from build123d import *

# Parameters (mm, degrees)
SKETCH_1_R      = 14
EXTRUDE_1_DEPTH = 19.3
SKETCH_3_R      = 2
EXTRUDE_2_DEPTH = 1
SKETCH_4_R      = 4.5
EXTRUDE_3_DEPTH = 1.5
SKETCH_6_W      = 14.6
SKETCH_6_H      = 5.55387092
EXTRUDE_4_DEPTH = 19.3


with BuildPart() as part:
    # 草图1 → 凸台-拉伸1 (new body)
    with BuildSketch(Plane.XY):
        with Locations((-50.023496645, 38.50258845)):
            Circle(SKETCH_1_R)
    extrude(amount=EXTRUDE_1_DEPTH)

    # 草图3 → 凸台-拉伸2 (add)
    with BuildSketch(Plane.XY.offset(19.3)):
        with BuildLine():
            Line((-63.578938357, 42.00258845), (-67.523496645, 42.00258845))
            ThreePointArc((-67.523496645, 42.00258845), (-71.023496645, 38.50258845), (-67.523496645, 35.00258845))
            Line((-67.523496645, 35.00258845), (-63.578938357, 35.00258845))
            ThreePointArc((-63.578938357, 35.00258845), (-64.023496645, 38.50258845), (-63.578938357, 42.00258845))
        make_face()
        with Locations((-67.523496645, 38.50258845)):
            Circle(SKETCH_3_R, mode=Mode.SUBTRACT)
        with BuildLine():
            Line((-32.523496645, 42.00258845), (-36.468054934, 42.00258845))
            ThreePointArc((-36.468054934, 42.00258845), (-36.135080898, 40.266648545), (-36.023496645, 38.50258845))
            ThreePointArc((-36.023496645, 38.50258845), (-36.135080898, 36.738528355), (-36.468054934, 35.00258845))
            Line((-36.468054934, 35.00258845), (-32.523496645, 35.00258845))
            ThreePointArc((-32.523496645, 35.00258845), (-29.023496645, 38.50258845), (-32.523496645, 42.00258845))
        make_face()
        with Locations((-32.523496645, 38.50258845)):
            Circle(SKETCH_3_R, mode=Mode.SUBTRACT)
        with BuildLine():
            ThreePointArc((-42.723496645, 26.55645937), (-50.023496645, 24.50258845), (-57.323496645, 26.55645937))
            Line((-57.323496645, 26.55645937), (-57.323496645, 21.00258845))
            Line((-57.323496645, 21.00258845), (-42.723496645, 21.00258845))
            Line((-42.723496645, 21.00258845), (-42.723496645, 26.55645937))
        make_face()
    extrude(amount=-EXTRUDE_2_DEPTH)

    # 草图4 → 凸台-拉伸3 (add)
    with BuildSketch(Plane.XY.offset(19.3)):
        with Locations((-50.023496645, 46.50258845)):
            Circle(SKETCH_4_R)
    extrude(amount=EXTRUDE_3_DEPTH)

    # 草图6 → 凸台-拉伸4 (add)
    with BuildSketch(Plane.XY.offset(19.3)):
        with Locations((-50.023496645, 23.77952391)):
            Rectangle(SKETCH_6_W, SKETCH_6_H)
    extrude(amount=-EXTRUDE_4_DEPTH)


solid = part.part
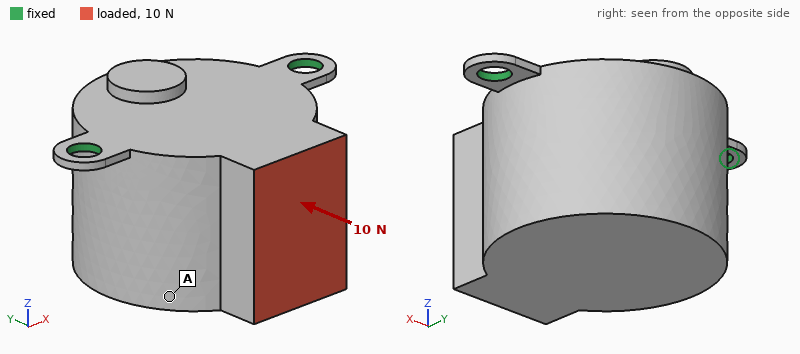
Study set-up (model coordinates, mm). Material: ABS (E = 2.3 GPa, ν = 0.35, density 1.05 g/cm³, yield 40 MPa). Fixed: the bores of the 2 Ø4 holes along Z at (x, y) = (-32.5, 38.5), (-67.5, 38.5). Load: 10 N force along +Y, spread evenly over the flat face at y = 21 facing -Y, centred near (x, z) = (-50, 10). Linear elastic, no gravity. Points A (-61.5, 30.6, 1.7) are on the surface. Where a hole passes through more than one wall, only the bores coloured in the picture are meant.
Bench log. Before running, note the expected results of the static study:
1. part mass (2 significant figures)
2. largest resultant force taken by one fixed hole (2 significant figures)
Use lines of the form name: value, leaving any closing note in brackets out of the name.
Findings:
part mass: 14 g
largest resultant force taken by one fixed hole: 5.0 N
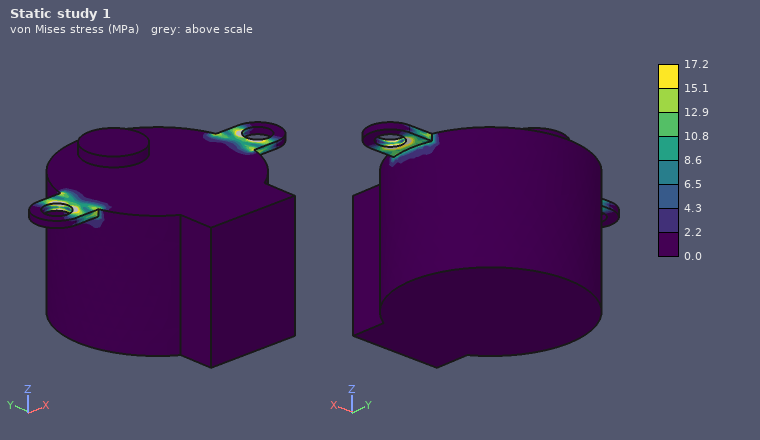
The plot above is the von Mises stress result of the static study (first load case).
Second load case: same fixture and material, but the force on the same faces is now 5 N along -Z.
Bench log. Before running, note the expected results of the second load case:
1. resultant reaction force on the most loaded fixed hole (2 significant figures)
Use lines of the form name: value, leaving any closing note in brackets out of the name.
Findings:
resultant reaction force on the most loaded fixed hole: 3.0 N
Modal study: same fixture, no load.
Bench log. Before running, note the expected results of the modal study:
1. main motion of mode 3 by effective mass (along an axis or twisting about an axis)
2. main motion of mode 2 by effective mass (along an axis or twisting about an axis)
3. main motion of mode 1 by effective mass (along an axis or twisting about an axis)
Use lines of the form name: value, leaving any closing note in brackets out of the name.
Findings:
main motion of mode 3 by effective mass: along X
main motion of mode 2 by effective mass: along Z
main motion of mode 1 by effective mass: along Y
